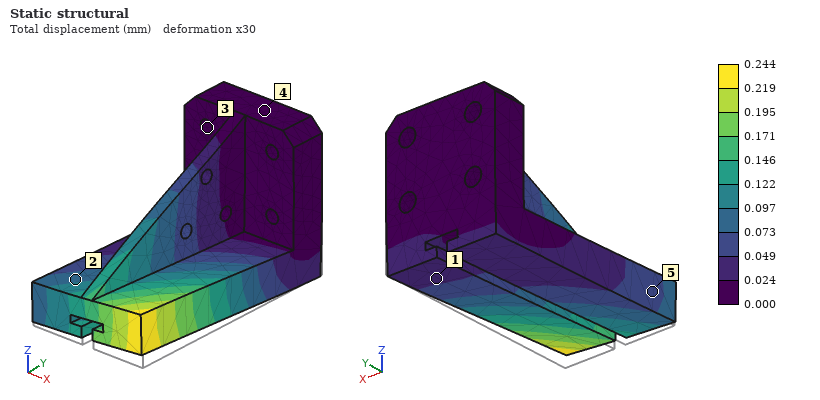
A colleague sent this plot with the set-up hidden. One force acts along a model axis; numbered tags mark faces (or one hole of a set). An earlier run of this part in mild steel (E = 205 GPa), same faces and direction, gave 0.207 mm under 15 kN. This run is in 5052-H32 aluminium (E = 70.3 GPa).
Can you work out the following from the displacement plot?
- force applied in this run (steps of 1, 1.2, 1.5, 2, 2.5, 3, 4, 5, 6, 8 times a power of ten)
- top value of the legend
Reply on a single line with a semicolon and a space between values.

6 kN; 0.244 mm
